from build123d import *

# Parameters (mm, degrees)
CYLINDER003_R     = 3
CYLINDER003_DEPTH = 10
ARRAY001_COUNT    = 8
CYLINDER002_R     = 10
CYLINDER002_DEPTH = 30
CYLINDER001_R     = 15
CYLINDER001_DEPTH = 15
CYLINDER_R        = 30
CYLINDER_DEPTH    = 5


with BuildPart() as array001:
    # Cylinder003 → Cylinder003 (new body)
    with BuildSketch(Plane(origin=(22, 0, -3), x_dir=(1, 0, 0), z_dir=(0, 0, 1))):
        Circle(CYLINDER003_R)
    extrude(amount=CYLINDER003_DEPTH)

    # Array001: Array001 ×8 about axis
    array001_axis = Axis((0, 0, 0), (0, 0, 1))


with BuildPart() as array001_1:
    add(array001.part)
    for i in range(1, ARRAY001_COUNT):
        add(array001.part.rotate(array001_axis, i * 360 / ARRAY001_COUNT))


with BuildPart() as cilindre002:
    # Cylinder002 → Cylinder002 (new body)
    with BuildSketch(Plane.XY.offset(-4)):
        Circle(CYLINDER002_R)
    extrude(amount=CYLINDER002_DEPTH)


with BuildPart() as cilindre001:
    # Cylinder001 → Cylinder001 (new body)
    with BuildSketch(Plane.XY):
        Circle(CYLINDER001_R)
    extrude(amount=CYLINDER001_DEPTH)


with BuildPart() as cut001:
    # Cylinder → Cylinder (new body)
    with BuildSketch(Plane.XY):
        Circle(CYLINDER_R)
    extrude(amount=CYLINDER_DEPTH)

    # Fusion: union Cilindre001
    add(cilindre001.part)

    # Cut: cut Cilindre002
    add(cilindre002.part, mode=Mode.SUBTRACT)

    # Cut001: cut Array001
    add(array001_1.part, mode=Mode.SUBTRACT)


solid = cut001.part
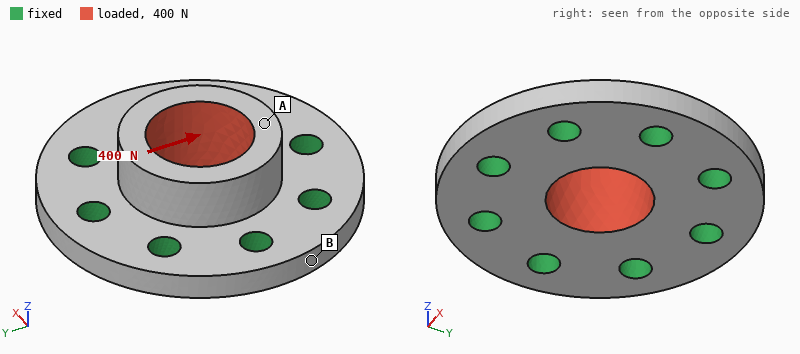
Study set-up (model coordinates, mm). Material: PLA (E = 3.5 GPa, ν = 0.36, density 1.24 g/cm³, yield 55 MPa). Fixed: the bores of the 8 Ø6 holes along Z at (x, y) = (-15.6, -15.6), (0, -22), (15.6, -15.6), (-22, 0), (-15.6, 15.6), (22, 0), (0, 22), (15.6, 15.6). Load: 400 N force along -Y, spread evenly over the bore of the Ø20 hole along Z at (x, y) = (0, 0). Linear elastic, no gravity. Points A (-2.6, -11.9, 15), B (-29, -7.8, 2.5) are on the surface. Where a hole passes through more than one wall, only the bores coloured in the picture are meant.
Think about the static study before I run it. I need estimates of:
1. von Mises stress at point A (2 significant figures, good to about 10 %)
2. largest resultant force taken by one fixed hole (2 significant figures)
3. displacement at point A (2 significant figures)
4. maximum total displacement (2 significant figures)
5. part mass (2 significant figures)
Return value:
1.3 MPa
80 N
13 µm
14 µm
19 g
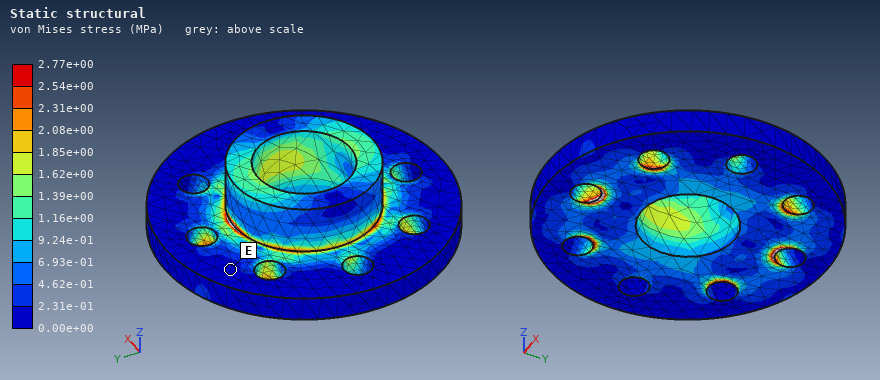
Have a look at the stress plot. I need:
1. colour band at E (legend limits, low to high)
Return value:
0.00e+00 to 2.31e-01 MPa
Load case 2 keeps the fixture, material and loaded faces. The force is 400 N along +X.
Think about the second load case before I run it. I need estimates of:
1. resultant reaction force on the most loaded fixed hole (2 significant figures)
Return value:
80 N
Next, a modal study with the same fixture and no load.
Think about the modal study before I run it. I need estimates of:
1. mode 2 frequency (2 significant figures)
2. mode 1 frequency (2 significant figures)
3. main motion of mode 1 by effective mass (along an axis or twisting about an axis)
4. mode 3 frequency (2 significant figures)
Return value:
12 kHz
11 kHz
along Z
12 kHz
